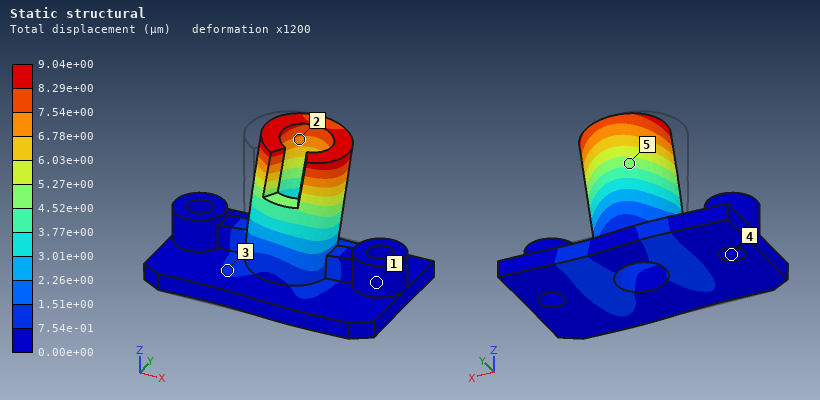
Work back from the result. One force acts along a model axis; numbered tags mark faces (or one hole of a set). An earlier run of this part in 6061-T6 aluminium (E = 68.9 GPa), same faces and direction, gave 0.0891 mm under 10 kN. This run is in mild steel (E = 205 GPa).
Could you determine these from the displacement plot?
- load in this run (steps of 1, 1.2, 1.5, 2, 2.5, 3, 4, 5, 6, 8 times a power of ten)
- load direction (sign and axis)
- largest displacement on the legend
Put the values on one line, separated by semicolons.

3 kN; +X; 9.04e+00 µm
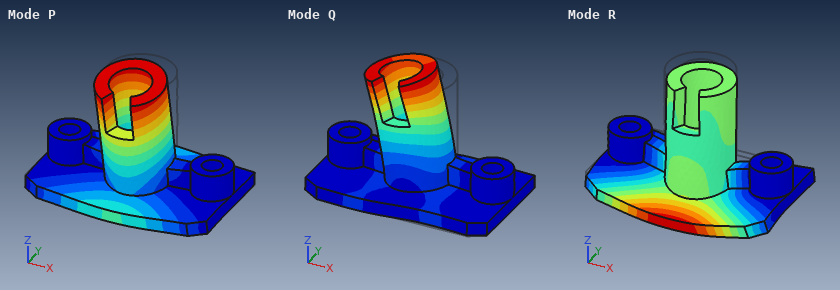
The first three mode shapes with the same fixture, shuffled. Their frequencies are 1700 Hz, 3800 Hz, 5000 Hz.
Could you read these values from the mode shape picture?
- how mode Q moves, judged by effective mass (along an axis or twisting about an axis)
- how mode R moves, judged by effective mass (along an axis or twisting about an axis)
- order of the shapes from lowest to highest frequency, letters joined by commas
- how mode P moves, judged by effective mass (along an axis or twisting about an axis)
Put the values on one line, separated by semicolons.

along X; along Z; P, Q, R; along Y
